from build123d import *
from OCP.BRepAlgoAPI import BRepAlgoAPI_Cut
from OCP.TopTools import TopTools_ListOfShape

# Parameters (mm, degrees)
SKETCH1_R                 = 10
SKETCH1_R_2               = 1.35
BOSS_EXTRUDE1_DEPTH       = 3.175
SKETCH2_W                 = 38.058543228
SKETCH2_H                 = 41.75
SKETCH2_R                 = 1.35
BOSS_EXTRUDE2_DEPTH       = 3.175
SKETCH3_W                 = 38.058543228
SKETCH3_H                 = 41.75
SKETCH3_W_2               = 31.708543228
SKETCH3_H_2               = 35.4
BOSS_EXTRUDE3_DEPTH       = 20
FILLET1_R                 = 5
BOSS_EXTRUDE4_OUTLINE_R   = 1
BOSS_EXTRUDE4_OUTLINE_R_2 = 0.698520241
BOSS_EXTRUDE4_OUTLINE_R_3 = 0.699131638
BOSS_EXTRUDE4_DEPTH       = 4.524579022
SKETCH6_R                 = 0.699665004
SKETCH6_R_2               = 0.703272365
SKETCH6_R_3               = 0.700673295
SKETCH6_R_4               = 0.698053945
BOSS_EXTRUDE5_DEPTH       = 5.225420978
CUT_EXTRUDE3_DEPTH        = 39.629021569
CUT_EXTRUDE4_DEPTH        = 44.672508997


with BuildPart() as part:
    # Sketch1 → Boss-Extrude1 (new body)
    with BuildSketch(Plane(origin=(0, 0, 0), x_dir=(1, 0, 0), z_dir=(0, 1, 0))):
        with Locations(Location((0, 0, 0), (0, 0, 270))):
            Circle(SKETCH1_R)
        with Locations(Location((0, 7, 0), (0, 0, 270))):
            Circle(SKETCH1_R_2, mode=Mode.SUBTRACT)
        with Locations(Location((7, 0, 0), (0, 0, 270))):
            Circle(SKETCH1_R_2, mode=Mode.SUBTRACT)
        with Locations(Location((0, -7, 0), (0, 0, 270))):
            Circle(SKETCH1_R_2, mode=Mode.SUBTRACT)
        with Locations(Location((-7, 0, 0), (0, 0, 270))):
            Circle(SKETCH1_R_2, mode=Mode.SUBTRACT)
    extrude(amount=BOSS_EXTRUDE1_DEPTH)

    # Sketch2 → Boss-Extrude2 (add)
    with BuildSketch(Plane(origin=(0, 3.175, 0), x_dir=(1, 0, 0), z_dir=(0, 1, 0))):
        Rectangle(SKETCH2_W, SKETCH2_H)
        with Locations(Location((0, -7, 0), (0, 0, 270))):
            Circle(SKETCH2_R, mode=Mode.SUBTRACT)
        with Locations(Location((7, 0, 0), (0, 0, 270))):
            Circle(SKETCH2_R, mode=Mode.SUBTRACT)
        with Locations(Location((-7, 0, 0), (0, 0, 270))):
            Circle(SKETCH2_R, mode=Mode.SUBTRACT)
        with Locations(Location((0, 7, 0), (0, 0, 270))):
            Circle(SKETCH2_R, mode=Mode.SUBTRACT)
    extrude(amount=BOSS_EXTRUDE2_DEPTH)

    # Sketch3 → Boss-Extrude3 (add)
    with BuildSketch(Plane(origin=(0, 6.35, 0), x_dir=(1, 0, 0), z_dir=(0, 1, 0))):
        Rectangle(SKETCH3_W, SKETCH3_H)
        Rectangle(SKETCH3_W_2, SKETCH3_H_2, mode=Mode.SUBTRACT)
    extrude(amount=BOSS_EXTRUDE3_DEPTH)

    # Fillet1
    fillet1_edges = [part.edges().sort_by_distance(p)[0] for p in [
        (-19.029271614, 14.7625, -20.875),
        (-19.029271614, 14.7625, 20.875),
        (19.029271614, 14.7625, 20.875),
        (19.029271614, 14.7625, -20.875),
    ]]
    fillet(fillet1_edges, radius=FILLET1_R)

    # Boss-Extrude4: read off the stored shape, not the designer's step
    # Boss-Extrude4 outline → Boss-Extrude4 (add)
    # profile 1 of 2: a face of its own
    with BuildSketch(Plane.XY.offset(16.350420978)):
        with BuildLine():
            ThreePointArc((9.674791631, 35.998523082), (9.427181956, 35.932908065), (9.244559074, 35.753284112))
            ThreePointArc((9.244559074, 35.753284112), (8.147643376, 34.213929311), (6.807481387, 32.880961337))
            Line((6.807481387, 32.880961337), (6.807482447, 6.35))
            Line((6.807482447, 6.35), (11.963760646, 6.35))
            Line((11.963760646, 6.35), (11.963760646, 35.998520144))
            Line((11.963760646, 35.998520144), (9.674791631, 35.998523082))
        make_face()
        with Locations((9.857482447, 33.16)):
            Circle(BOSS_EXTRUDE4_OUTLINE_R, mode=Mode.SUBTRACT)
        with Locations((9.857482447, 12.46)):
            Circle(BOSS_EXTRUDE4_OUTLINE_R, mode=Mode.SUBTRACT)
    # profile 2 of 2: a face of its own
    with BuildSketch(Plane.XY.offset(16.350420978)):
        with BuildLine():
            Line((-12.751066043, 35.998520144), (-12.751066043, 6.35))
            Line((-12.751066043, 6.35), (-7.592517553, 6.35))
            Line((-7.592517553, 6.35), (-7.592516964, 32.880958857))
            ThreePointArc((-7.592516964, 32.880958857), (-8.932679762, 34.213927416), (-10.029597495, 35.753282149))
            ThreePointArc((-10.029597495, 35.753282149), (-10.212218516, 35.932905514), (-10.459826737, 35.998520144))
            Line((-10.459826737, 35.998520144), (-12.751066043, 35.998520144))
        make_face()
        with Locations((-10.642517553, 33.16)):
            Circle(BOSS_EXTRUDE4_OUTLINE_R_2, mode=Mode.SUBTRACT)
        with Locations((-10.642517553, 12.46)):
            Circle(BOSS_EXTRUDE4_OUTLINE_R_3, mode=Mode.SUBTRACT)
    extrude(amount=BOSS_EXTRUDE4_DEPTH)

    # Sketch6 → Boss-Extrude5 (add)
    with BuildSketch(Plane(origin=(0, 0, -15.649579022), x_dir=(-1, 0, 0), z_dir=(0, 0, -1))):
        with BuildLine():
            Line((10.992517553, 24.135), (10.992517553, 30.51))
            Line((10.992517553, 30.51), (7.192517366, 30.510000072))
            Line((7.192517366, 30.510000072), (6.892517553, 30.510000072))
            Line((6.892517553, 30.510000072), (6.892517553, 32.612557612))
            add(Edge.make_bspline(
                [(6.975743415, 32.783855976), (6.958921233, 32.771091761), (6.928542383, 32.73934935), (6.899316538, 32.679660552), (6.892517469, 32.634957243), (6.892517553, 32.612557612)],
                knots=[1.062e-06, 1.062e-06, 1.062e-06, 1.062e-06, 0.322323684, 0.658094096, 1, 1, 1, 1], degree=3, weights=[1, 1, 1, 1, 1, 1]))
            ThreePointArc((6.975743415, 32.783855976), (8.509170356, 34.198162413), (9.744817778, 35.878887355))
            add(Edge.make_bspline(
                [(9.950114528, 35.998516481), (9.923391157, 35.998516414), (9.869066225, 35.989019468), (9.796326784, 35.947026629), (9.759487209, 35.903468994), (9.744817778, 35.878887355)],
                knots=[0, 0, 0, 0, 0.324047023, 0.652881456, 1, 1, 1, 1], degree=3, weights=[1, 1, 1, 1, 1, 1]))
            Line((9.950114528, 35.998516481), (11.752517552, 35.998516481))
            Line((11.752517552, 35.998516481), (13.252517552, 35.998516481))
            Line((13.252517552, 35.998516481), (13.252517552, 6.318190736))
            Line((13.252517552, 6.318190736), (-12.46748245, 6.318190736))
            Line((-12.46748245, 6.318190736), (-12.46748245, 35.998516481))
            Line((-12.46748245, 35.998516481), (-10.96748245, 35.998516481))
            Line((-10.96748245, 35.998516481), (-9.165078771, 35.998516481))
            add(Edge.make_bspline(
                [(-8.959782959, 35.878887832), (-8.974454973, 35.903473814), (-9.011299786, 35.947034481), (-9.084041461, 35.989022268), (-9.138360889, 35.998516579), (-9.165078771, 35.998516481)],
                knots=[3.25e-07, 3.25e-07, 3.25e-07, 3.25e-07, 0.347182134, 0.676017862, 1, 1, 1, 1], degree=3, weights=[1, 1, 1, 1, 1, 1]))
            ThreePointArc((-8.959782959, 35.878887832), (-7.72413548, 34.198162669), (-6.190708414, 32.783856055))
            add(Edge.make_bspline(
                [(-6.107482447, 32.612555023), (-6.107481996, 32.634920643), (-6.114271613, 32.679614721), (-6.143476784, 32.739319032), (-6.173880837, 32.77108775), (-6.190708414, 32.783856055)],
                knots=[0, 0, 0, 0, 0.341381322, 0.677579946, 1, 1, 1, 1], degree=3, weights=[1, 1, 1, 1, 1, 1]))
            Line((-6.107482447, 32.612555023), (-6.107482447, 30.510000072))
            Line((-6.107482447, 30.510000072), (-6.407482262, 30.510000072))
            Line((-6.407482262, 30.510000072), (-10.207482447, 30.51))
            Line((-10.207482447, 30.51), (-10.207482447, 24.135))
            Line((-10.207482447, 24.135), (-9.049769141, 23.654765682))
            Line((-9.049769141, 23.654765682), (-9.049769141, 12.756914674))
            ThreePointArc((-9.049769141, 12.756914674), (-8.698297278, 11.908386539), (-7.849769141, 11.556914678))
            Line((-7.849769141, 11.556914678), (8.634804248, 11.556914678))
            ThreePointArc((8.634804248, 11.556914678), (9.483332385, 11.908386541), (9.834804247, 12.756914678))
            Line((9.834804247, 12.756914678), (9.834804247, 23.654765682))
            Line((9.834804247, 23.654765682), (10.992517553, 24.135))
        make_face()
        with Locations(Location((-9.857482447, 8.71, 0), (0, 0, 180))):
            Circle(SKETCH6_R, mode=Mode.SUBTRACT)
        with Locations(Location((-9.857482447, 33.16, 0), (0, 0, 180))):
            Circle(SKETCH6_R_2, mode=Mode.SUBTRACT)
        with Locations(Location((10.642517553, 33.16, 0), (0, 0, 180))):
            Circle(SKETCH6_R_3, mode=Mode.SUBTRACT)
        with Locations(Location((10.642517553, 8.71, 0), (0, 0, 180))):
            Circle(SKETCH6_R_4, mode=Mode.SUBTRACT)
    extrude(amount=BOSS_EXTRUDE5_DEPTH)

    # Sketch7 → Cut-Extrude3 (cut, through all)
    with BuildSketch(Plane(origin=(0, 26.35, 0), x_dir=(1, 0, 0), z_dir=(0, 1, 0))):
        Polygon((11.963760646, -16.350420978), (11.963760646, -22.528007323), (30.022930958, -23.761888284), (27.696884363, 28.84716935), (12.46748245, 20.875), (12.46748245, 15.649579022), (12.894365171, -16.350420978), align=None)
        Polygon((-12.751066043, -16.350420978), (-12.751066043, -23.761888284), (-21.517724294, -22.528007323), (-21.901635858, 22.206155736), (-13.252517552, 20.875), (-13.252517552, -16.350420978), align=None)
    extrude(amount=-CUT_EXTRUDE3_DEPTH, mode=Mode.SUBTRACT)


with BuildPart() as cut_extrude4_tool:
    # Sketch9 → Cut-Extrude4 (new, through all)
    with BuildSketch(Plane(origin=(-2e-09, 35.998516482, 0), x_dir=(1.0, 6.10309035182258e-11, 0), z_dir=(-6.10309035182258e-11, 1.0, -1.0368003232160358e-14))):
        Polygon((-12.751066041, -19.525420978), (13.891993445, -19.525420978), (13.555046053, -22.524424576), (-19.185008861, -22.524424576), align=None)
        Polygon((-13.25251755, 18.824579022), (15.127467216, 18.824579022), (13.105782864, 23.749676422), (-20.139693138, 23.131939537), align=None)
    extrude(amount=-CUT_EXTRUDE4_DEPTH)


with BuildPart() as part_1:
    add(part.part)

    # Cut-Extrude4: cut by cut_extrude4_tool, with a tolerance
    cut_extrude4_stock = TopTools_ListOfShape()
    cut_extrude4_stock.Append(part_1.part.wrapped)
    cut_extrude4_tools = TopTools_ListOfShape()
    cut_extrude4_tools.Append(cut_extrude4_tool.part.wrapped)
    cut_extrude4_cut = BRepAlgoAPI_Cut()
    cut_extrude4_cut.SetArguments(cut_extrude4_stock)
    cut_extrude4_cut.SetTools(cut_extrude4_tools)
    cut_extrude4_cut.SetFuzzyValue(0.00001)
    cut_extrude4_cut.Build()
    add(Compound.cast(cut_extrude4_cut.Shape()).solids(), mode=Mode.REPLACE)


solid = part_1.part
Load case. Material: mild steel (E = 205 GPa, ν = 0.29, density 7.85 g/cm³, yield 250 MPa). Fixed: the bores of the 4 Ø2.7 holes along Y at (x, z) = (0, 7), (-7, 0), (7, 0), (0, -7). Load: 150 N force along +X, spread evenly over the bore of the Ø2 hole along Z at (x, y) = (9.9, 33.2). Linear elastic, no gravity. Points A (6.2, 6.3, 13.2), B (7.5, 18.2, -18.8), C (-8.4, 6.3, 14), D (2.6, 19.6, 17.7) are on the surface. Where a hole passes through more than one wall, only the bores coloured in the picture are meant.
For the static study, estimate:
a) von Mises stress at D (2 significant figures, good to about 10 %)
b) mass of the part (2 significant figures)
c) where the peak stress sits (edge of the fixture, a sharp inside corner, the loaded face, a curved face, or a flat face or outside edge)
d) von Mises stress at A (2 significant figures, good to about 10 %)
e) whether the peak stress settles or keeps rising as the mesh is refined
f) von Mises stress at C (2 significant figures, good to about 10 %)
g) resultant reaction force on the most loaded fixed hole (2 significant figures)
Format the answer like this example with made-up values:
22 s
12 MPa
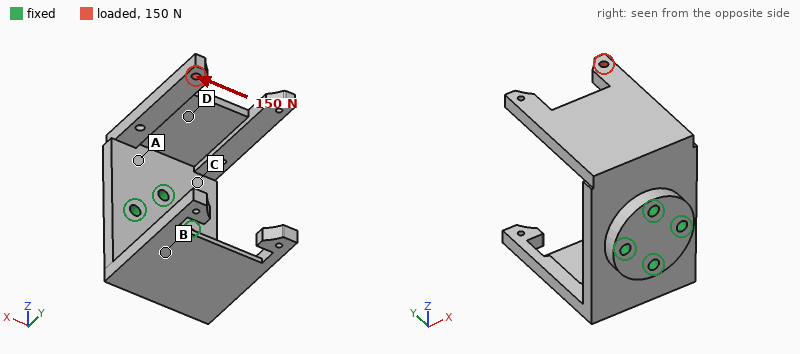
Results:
30 MPa
53 g
edge of the fixture
52 MPa
keeps rising
46 MPa
160 N
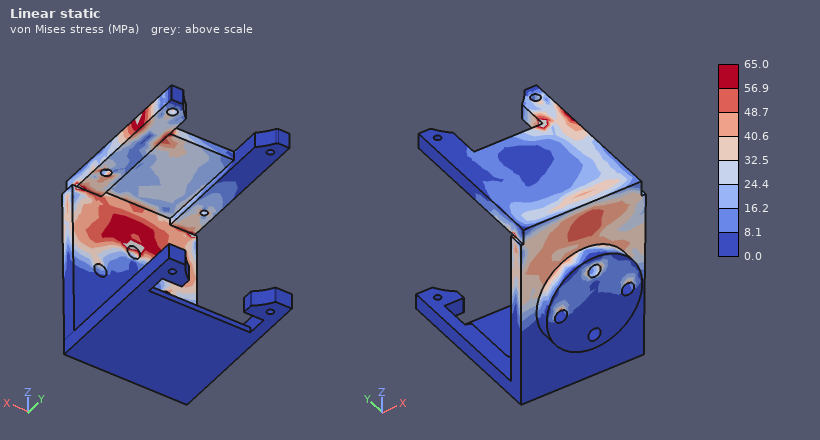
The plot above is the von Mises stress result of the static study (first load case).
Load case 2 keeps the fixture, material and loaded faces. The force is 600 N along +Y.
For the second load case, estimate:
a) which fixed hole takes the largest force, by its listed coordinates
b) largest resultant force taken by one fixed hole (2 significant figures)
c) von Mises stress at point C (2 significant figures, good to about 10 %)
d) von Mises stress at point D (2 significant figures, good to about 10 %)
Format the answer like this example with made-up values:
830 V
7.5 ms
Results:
(0, 7)
800 N
85 MPa
11 MPa
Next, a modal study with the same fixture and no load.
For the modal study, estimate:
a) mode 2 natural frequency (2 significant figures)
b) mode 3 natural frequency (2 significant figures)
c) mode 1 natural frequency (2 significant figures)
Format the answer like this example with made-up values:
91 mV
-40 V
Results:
2500 Hz
3300 Hz
2300 Hz
